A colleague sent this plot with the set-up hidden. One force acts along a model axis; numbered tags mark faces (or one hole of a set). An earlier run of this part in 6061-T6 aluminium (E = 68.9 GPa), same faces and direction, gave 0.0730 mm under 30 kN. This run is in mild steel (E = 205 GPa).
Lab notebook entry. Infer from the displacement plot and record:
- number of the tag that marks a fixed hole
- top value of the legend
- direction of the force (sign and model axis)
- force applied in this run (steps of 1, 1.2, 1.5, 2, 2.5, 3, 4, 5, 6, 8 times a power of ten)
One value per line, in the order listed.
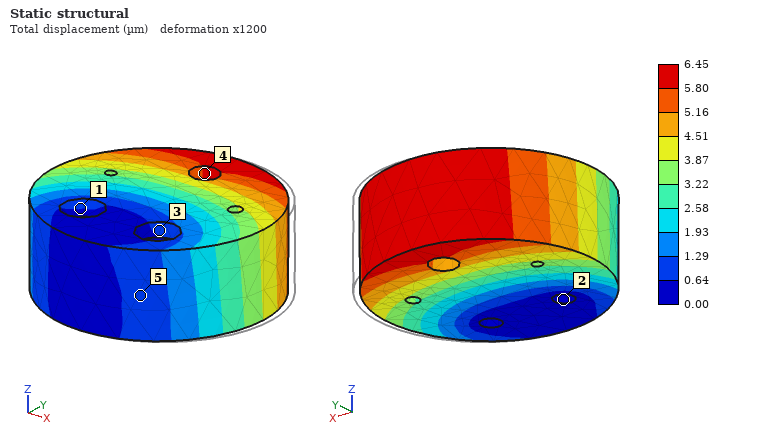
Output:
2
6.45 µm
-X
8 kN
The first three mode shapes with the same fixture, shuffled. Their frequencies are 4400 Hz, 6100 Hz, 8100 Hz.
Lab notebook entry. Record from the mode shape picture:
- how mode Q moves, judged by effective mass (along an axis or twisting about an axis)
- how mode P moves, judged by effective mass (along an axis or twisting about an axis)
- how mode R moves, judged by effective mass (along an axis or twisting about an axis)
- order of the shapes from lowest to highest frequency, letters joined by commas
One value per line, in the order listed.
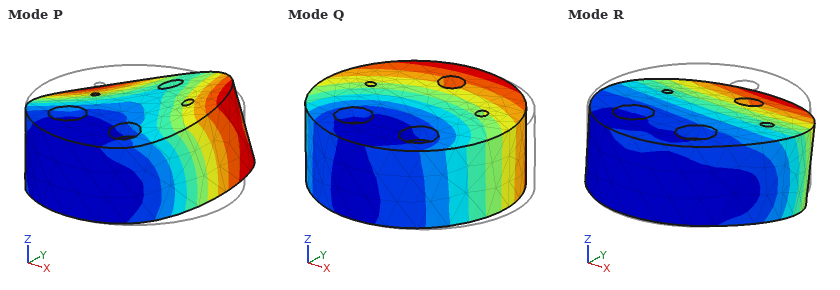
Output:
along X
twisting about Y
along Z
R, Q, P
